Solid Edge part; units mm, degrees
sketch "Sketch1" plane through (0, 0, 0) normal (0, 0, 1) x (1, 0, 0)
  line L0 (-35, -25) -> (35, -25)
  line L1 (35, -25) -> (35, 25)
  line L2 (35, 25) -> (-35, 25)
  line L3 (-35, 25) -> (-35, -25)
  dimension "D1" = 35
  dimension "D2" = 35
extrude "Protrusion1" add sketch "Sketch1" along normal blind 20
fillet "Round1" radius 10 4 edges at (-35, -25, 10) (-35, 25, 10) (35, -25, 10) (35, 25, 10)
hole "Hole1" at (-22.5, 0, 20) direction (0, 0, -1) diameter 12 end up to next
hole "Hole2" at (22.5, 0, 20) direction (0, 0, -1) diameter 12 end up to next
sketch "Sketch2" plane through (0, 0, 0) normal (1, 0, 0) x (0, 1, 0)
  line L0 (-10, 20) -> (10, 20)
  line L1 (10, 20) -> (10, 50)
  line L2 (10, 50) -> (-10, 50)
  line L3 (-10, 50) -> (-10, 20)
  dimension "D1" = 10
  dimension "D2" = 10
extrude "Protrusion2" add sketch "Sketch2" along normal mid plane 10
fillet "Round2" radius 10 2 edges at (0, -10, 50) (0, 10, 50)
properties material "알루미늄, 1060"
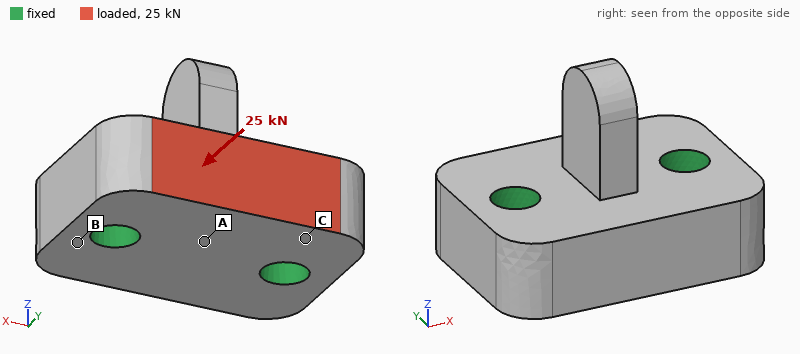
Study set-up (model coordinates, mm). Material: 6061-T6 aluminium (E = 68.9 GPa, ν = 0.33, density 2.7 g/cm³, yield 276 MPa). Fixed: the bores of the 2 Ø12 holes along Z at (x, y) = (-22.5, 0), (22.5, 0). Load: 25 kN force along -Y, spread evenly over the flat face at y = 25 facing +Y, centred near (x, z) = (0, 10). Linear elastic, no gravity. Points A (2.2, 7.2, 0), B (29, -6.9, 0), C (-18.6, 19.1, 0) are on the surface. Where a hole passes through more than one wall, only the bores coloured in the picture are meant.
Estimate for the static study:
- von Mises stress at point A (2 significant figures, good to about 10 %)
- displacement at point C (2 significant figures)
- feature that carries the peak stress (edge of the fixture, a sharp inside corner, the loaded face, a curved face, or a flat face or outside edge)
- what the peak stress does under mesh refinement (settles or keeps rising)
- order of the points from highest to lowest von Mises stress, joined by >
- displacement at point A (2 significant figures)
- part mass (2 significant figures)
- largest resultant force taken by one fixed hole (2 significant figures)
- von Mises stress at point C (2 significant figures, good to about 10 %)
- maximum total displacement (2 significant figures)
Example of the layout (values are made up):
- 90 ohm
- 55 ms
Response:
- 14 MPa
- 6.1 µm
- edge of the fixture
- keeps rising
- C > A > B
- 6.7 µm
- 190 g
- 13 kN
- 25 MPa
- 12 µm
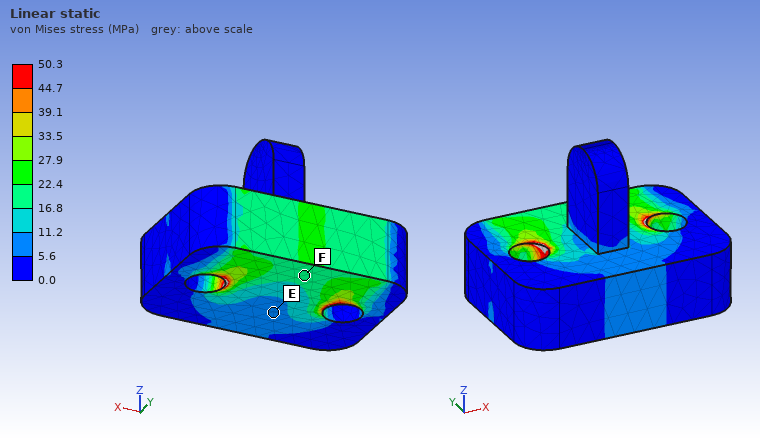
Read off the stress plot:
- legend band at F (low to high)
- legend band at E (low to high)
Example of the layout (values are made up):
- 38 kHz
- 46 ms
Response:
- 16.8 to 22.4 MPa
- 5.6 to 11.2 MPa
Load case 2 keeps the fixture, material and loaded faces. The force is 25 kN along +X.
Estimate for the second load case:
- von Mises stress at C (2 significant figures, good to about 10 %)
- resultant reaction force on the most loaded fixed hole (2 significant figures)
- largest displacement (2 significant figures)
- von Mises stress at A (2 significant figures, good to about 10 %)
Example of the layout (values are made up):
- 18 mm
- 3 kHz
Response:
- 33 MPa
- 16 kN
- 22 µm
- 29 MPa
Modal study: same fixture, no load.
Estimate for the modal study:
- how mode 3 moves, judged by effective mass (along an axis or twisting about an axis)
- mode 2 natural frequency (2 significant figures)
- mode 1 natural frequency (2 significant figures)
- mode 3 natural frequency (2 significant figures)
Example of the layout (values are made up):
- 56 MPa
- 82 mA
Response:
- along Z
- 11 kHz
- 8100 Hz
- 20 kHz
